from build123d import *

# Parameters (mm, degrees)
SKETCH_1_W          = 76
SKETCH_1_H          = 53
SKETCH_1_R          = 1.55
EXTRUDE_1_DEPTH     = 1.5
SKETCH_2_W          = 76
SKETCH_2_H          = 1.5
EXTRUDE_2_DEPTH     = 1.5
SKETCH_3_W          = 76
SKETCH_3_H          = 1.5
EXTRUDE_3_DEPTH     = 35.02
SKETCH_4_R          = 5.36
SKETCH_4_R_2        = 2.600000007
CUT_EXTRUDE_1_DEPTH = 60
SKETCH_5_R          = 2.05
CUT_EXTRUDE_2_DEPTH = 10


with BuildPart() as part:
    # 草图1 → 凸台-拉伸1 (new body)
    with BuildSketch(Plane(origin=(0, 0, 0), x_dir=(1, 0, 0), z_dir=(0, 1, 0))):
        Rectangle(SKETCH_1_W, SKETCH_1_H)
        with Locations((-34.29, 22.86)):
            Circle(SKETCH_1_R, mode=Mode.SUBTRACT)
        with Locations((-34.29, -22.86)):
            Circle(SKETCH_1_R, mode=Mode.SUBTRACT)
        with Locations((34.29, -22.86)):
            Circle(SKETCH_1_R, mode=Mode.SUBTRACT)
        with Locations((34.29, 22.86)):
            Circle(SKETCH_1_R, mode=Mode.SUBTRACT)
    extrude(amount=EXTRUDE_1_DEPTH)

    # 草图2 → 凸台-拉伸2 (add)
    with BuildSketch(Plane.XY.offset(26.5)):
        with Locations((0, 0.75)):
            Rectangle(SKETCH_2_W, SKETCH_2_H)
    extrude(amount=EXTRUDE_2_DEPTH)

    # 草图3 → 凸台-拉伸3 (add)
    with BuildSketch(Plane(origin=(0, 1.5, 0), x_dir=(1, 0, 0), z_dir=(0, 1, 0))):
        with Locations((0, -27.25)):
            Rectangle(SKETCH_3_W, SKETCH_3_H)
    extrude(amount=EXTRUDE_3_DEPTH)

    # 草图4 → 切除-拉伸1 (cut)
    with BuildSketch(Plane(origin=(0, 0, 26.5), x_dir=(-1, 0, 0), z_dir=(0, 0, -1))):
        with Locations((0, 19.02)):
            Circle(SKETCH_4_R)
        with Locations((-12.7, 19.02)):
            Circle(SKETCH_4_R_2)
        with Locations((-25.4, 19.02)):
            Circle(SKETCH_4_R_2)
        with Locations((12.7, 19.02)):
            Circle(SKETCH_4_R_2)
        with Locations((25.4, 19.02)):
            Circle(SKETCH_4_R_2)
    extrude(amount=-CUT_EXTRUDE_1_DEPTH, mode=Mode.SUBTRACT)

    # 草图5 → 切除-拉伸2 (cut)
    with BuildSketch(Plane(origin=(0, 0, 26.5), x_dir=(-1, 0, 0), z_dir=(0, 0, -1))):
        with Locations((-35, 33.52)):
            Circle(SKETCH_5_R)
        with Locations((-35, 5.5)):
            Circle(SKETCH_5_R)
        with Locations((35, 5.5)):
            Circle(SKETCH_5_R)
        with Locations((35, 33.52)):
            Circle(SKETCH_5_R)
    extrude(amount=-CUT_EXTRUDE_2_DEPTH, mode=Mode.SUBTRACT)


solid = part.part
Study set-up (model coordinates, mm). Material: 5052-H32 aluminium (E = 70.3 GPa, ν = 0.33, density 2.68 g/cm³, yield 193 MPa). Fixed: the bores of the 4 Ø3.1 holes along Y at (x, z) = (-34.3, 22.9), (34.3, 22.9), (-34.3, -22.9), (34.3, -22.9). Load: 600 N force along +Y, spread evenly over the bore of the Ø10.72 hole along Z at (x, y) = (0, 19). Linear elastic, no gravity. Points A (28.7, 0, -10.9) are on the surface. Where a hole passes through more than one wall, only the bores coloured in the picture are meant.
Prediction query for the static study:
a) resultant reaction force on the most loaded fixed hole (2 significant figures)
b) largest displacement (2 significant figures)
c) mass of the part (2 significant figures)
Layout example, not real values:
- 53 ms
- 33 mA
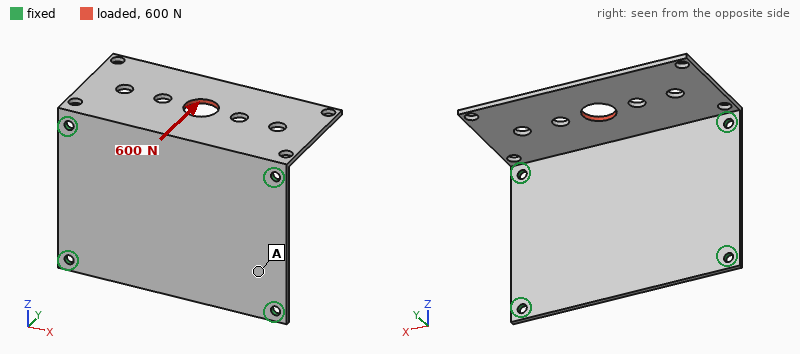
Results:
- 360 N
- 0.19 mm
- 26 g
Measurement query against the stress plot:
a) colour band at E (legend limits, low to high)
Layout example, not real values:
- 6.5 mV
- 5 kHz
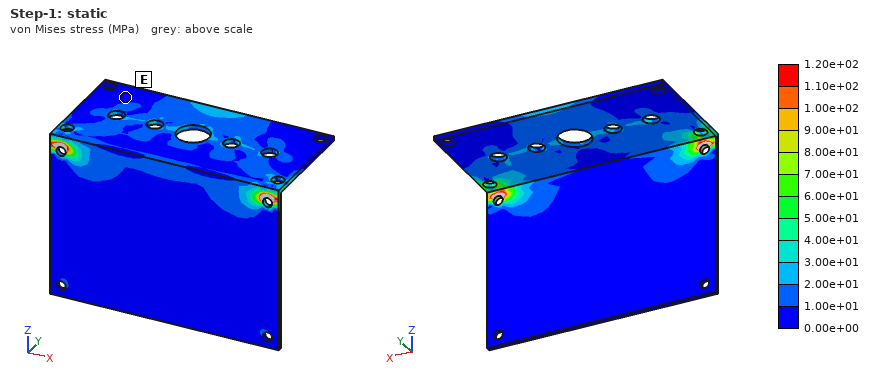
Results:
- 0.00e+00 to 1.00e+01 MPa
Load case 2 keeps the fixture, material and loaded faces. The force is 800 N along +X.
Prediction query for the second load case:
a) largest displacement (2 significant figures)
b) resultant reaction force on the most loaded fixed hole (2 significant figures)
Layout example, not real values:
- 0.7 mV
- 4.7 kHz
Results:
- 90 µm
- 410 N
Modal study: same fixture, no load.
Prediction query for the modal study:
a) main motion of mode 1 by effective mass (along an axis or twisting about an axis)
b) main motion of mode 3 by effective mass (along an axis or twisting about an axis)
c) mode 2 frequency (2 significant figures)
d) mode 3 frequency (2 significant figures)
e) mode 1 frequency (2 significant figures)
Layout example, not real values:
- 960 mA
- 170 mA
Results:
- along Z
- along Y
- 1300 Hz
- 1700 Hz
- 730 Hz
